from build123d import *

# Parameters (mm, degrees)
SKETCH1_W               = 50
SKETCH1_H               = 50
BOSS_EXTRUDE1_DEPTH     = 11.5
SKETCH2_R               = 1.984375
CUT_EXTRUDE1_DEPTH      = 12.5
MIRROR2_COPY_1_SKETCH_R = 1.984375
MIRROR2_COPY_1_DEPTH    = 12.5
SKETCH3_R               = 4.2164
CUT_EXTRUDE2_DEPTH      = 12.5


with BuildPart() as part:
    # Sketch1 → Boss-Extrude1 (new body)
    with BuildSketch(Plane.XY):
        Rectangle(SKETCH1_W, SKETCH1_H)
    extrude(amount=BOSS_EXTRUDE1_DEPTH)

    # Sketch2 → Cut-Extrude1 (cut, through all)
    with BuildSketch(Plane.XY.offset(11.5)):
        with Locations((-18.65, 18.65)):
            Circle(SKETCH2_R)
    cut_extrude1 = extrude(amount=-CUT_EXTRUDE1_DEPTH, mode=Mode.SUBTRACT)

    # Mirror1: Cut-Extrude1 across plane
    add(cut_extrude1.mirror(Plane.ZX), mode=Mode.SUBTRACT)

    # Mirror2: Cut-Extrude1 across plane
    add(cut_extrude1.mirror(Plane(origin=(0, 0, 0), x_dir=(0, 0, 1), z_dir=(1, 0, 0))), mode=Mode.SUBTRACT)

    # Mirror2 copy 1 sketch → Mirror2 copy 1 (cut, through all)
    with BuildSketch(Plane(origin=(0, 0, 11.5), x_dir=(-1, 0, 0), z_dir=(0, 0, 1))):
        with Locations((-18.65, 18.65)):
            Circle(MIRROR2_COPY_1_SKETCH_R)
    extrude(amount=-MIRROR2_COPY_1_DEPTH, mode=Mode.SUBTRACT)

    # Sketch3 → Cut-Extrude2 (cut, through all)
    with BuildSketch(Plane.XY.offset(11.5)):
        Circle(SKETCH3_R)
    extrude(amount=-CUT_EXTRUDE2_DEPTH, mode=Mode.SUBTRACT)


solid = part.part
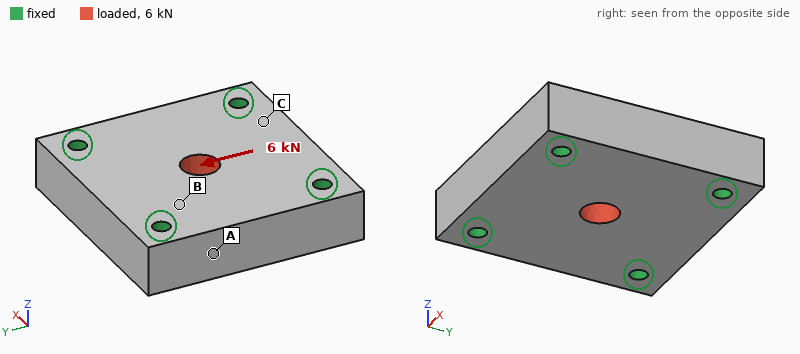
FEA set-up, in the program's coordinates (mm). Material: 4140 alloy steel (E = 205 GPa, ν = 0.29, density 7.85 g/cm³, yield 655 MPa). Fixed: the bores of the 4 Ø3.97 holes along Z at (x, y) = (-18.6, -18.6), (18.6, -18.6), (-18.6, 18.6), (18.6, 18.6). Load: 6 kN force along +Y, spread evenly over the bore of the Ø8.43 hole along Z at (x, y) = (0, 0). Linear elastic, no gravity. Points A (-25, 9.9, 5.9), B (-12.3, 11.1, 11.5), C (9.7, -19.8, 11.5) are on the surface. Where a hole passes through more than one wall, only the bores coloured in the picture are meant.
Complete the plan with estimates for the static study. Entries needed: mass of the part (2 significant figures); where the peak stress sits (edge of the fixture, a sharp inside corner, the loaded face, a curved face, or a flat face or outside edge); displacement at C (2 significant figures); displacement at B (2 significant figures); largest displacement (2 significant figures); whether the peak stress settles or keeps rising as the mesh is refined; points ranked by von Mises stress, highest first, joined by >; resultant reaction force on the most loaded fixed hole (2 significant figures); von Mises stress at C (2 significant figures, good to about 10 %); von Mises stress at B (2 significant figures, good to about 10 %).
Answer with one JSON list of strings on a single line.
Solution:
["220 g", "edge of the fixture", "0.78 µm", "0.64 µm", "1.9 µm", "keeps rising", "B > C > A", "1.7 kN", "6.7 MPa", "12 MPa"]
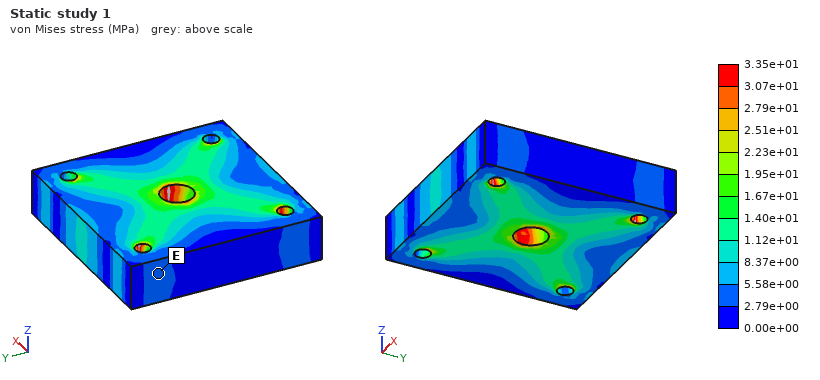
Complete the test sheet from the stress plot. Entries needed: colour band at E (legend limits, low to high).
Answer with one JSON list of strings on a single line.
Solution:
["2.79e+00 to 5.58e+00 MPa"]
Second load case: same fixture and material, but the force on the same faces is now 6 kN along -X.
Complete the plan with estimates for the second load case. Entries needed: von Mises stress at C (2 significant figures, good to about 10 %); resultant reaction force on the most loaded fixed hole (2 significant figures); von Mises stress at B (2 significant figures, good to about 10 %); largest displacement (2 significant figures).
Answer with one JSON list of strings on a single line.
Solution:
["5.5 MPa", "1.7 kN", "13 MPa", "1.9 µm"]
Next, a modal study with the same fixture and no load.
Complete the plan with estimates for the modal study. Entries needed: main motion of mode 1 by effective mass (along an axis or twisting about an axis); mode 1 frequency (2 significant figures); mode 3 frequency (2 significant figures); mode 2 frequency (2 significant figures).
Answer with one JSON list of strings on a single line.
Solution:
["along Z", "21 kHz", "31 kHz", "31 kHz"]
